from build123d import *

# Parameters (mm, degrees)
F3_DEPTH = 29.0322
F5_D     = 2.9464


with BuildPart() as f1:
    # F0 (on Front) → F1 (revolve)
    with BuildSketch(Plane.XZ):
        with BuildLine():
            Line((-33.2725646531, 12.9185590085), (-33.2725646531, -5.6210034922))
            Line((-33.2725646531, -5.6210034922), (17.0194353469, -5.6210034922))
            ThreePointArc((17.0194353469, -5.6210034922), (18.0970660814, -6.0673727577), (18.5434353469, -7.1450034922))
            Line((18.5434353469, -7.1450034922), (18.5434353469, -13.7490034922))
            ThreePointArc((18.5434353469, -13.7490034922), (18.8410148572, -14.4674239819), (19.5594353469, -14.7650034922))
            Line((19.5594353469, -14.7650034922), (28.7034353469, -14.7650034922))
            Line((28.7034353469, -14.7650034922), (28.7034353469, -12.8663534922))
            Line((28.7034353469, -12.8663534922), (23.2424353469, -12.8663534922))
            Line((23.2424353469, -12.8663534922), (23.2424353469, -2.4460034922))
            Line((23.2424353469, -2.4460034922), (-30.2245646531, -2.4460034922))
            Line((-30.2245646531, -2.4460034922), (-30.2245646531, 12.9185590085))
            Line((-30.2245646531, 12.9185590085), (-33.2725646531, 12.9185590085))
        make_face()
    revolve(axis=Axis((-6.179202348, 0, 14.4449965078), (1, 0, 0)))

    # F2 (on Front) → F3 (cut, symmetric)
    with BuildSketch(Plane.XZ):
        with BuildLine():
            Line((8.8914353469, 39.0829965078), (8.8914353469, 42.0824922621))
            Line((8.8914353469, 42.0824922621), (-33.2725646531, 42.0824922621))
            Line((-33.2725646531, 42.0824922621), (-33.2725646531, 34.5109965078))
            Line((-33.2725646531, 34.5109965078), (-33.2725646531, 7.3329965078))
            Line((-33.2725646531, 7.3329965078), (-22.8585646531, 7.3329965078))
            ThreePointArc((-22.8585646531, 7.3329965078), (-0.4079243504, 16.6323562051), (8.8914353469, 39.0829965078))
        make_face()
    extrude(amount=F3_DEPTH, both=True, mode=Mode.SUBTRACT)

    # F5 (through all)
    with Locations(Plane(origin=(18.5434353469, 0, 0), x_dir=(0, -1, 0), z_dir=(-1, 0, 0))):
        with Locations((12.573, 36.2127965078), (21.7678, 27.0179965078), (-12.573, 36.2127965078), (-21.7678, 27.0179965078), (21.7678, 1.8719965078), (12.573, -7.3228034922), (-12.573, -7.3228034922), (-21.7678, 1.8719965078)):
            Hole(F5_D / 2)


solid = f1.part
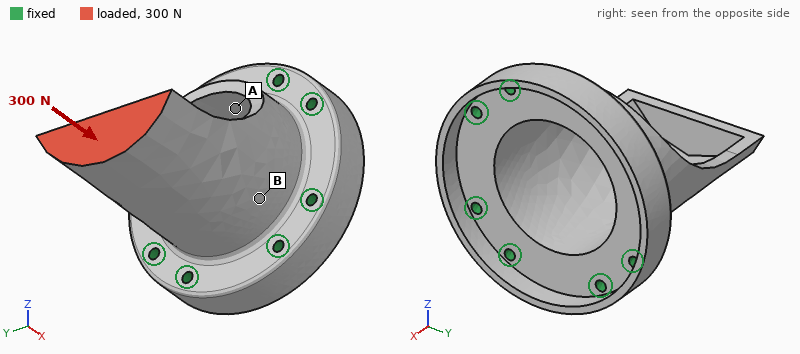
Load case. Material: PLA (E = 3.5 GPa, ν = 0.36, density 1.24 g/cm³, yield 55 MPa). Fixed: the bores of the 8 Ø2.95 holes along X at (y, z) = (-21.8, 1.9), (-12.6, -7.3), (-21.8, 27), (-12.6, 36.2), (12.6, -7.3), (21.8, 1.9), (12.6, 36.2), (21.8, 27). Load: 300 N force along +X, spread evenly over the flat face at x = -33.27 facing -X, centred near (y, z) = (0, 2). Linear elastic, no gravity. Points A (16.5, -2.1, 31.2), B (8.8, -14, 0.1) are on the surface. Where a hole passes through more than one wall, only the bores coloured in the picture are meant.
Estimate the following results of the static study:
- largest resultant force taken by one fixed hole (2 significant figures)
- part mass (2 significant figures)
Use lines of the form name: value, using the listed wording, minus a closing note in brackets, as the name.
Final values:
largest resultant force taken by one fixed hole: 79 N
part mass: 27 g
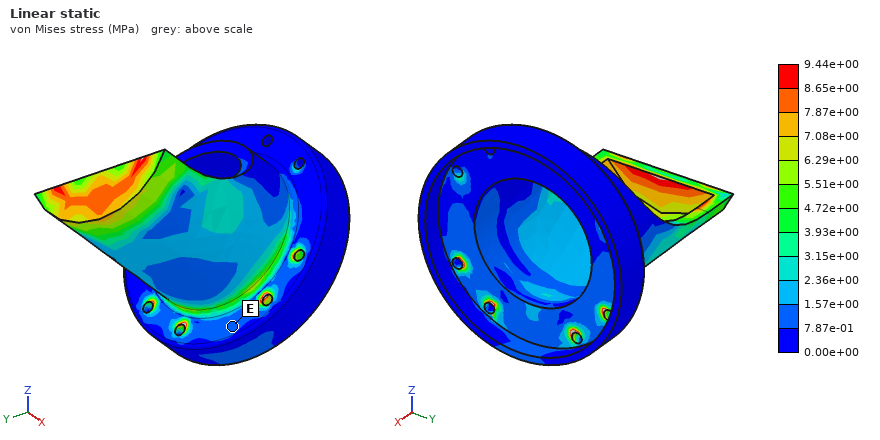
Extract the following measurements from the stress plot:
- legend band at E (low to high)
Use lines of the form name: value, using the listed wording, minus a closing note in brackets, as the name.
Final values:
legend band at E: 7.87e-01 to 1.57e+00 MPa
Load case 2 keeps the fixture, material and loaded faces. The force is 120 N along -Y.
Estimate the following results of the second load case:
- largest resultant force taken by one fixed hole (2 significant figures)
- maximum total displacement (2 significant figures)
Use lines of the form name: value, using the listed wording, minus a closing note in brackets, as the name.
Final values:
largest resultant force taken by one fixed hole: 120 N
maximum total displacement: 0.70 mm
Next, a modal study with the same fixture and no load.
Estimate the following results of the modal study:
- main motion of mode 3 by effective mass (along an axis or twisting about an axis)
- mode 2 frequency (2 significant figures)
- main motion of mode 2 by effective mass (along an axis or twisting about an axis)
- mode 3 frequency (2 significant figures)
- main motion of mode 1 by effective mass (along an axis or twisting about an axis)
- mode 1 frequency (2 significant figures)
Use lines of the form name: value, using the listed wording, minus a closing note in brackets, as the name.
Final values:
main motion of mode 3 by effective mass: along Y
mode 2 frequency: 1600 Hz
main motion of mode 2 by effective mass: along Z
mode 3 frequency: 3200 Hz
main motion of mode 1 by effective mass: along Y
mode 1 frequency: 1400 Hz
